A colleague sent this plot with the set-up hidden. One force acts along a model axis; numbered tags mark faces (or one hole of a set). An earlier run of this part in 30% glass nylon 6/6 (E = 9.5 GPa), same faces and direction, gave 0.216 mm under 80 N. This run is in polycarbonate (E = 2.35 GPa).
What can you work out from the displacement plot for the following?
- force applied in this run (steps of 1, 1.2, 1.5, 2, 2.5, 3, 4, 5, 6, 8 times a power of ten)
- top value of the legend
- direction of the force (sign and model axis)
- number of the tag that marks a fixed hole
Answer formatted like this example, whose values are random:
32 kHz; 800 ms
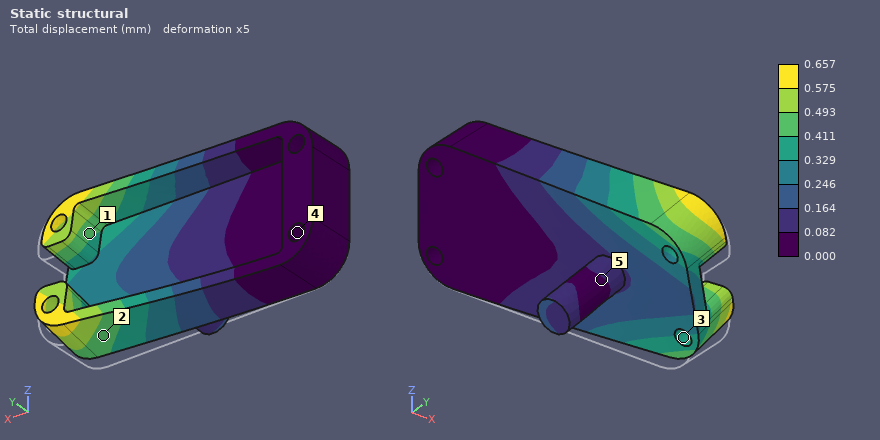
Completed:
60 N; 0.657 mm; +Z; 4
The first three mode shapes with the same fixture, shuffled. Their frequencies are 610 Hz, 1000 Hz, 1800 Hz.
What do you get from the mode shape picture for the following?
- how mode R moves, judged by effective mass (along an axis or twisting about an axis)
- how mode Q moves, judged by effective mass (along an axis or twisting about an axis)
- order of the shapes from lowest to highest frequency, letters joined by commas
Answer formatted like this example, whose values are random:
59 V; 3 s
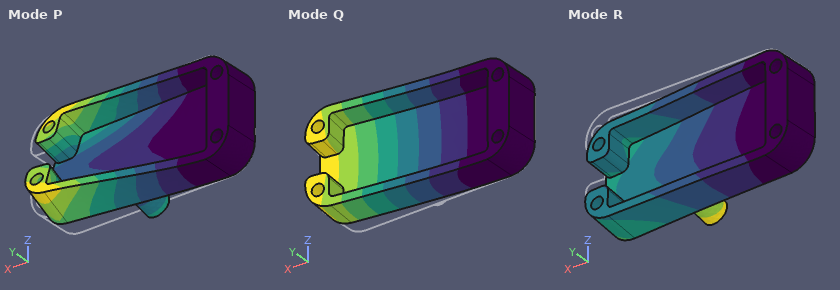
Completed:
along Z; along Y; Q, P, R
